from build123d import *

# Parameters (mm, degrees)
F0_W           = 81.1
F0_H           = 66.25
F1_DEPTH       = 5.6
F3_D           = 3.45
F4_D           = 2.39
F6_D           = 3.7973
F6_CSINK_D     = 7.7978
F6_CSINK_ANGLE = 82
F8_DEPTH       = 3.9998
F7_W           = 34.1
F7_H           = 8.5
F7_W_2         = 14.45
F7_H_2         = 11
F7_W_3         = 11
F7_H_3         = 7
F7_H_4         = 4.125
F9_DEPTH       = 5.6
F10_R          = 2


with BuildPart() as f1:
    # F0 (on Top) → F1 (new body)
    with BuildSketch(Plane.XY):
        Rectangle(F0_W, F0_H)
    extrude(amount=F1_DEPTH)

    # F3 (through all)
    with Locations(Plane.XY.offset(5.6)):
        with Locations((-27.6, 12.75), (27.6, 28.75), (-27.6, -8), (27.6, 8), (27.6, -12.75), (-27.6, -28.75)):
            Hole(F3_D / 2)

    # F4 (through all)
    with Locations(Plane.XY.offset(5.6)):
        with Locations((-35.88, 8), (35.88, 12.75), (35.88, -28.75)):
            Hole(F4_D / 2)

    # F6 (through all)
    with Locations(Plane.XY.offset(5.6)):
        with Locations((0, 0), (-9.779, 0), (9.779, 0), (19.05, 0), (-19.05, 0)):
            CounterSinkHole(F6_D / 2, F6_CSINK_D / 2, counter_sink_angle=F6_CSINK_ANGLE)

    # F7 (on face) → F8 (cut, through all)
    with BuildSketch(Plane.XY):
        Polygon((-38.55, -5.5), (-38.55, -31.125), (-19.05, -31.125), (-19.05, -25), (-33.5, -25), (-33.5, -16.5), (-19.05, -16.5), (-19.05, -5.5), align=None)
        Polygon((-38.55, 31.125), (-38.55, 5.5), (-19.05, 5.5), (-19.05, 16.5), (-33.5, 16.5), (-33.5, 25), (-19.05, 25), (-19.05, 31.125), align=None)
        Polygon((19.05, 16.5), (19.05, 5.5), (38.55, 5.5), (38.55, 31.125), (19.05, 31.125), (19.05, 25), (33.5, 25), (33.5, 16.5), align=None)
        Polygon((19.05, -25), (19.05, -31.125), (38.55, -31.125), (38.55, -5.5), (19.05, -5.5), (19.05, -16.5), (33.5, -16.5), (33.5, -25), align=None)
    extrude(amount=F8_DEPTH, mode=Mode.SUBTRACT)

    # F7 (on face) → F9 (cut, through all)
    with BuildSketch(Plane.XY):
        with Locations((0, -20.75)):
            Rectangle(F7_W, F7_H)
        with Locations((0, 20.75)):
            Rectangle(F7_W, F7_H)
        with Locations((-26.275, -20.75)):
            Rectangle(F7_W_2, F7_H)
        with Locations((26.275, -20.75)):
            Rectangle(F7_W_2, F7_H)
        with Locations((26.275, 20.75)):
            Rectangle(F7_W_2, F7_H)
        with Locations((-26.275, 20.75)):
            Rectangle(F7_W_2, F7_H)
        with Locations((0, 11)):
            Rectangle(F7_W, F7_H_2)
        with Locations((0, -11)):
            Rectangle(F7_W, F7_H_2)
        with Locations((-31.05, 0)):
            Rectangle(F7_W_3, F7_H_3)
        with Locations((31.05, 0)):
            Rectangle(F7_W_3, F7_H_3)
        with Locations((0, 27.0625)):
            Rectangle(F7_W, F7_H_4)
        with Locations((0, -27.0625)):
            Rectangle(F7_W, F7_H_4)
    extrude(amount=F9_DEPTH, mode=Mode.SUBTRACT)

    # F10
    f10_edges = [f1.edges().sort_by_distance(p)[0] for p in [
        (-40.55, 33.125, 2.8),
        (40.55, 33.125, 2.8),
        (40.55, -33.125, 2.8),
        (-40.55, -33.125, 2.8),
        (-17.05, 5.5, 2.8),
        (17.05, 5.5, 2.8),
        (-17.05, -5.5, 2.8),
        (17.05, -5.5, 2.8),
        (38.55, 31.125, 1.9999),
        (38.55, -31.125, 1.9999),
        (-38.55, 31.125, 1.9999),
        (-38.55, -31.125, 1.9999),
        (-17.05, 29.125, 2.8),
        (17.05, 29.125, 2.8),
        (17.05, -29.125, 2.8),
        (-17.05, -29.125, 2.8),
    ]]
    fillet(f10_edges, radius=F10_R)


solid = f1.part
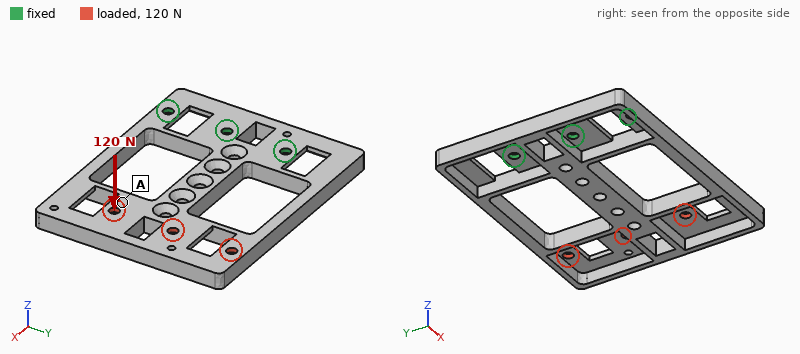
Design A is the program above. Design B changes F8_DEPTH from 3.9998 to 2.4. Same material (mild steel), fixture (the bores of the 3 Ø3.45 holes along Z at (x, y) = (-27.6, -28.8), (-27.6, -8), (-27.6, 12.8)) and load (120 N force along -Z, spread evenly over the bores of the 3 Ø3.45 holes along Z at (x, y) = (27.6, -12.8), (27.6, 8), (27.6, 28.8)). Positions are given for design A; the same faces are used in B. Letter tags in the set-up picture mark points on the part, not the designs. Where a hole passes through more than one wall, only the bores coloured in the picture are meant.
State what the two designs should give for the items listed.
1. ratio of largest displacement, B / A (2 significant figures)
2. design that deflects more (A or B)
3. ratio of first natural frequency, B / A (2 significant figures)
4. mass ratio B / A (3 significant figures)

0.57
A
1.2
1.21
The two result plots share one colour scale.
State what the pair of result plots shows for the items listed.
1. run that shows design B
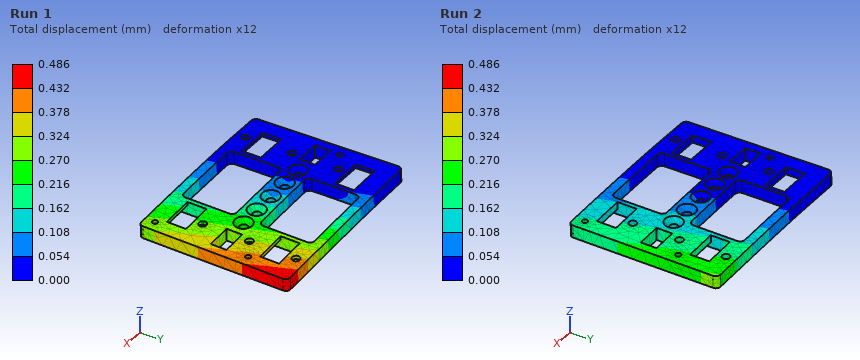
Run 2
